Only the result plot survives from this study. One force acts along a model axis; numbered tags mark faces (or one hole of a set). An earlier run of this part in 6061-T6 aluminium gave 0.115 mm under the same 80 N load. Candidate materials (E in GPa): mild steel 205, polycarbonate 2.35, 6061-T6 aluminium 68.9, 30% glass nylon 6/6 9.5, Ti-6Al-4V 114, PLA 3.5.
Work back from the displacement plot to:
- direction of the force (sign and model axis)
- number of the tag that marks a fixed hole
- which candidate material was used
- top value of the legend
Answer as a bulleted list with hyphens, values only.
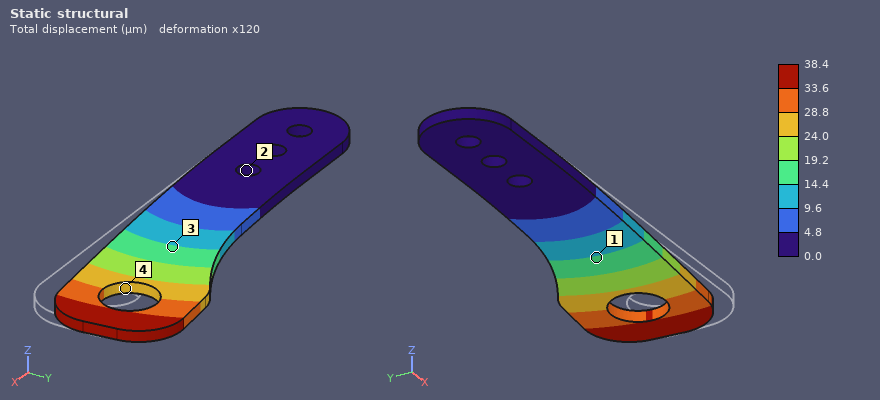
- +Y
- 2
- mild steel
- 38.4 µm
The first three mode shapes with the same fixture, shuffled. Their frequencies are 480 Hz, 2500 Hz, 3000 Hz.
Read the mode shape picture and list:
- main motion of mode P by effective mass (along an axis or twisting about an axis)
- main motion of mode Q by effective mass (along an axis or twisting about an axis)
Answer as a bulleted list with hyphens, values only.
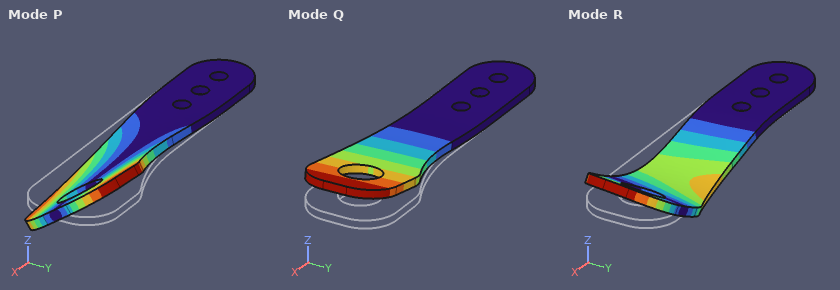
- twisting about X
- along Z
